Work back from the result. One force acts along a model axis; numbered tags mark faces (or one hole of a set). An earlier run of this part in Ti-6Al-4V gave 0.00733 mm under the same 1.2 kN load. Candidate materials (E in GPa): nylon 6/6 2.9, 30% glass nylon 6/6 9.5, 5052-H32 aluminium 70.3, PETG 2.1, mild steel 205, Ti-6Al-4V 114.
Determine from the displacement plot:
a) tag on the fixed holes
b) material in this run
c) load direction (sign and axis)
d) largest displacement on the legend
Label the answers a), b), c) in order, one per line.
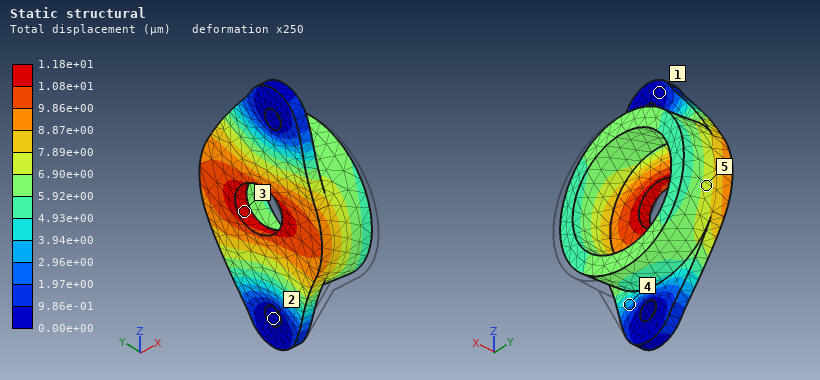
a) 2
b) 5052-H32 aluminium
c) +Y
d) 1.18e+01 µm
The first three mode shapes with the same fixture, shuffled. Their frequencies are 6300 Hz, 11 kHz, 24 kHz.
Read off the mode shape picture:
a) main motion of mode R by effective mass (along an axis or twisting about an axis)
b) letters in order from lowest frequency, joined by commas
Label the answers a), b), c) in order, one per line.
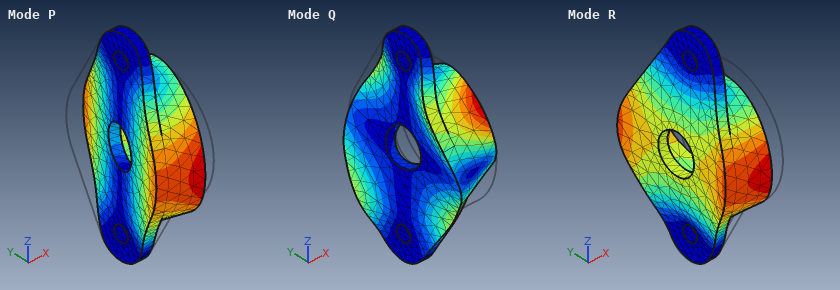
a) along X
b) P, R, Q
